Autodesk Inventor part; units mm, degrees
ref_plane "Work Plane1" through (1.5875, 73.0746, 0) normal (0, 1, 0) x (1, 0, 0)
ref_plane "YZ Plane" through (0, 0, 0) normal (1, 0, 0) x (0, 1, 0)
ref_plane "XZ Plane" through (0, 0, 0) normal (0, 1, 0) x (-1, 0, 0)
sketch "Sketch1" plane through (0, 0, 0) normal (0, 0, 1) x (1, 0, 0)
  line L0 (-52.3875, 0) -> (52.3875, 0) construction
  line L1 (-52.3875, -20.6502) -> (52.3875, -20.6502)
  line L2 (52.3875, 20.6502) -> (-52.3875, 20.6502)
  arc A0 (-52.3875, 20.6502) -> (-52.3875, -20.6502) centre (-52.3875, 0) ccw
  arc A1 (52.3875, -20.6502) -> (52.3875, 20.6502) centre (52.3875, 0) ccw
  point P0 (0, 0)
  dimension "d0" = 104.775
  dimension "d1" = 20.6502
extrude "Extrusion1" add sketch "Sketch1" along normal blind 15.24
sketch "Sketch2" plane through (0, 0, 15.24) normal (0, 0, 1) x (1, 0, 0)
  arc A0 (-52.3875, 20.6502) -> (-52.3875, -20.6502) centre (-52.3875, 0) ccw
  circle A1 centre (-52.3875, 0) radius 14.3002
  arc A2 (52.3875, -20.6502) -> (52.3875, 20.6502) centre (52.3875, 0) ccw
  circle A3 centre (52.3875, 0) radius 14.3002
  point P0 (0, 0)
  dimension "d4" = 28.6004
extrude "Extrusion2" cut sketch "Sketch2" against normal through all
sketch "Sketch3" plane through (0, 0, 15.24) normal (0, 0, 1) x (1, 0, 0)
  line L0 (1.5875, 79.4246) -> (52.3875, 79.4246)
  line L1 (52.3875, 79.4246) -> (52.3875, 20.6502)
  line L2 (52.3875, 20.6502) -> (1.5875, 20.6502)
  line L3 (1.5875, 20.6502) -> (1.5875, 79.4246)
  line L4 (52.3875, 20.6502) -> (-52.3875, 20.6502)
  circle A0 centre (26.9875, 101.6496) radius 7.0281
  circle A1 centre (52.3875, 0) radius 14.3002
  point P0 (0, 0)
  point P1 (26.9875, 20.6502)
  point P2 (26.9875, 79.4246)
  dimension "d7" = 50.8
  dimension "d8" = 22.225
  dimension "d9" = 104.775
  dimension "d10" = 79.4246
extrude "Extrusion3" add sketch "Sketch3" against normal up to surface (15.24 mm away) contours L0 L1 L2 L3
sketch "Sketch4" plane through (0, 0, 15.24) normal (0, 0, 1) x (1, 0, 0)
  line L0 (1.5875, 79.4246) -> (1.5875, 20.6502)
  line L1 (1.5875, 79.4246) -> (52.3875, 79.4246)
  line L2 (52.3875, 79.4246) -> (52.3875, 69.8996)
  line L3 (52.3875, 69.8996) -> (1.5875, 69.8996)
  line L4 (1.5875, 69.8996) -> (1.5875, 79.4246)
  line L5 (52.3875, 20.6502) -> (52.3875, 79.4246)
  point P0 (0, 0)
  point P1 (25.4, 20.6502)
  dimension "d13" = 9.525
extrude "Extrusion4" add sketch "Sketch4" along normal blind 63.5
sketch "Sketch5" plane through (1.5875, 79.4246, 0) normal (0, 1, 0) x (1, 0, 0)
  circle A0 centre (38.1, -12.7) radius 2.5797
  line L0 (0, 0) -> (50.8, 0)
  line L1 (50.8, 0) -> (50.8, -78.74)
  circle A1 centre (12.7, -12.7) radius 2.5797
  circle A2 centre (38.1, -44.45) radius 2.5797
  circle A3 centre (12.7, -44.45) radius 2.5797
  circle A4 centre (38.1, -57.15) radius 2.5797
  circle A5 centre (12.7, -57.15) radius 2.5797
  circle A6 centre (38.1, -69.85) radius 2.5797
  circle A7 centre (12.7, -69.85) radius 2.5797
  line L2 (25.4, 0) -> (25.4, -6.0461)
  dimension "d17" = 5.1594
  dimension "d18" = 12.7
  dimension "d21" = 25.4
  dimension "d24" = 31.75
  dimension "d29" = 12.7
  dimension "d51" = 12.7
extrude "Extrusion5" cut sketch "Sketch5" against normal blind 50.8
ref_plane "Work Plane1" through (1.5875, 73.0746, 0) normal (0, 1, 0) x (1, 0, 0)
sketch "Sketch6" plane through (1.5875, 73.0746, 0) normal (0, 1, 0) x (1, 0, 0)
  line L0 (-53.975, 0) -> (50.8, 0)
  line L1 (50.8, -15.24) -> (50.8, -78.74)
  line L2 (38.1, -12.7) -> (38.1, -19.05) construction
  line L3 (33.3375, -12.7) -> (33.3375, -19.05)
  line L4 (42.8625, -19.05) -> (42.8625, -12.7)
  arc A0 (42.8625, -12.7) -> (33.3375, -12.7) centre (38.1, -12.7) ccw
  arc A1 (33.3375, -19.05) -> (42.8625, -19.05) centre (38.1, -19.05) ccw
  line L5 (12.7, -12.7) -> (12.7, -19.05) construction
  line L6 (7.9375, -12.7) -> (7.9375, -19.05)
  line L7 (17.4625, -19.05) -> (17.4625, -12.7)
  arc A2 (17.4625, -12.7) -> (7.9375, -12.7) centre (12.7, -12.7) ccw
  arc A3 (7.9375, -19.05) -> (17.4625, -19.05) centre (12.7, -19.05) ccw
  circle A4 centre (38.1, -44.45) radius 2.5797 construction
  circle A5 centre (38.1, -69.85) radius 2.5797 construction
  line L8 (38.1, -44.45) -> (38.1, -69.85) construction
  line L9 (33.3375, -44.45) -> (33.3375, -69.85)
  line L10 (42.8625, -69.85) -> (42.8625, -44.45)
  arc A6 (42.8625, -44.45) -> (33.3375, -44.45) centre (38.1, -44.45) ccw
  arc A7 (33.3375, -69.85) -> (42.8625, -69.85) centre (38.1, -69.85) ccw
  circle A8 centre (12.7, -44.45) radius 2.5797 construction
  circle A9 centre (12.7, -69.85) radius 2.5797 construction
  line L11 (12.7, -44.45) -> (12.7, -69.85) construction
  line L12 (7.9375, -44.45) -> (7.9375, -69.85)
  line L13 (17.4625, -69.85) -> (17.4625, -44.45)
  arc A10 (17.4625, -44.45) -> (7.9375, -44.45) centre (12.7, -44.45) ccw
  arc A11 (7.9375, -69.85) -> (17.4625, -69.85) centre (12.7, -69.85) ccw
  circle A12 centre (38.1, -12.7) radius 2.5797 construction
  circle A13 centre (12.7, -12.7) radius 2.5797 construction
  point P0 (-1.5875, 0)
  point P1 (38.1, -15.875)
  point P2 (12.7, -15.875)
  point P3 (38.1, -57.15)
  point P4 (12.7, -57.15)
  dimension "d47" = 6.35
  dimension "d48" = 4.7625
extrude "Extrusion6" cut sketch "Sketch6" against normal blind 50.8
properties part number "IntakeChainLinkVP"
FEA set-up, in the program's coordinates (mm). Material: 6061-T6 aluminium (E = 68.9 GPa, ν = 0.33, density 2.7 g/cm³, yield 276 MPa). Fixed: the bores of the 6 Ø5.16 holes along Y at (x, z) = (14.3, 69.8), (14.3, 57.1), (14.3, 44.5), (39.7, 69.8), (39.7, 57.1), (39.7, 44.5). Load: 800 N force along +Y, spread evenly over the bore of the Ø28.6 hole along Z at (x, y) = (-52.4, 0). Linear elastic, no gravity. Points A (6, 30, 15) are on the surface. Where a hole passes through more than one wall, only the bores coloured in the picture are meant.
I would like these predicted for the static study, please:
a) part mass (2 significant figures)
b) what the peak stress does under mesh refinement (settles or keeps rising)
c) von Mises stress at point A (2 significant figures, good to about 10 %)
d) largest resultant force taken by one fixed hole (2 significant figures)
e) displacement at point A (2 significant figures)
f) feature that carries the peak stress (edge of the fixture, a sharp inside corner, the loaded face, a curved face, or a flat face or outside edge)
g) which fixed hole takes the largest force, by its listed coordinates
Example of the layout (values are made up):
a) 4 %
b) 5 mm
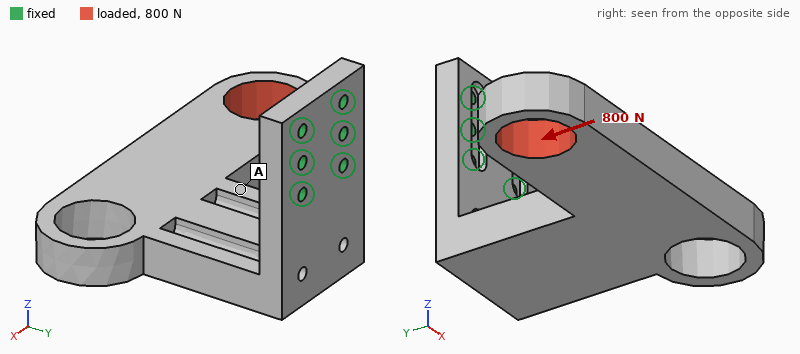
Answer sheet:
a) 360 g
b) keeps rising
c) 16 MPa
d) 3.3 kN
e) 0.30 mm
f) edge of the fixture
g) (14.3, 44.5)
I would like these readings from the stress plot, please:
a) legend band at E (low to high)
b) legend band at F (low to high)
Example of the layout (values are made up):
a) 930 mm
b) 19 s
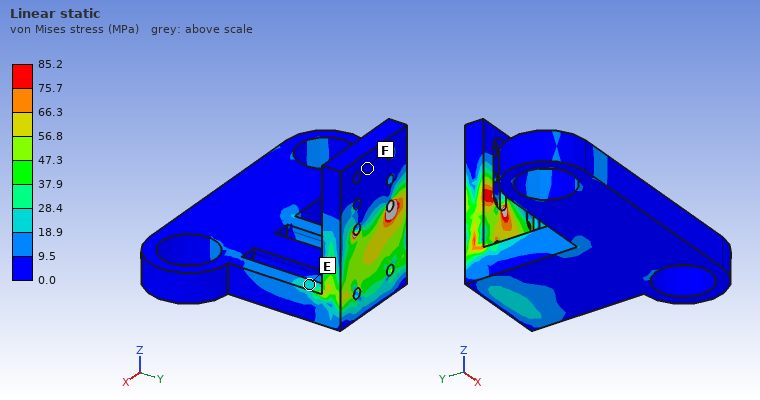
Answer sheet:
a) 18.9 to 28.4 MPa
b) 0.0 to 9.5 MPa
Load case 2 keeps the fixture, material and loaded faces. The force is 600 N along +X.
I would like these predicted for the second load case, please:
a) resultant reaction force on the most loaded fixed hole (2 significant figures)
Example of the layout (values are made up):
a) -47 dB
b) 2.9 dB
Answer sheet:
a) 1.9 kN
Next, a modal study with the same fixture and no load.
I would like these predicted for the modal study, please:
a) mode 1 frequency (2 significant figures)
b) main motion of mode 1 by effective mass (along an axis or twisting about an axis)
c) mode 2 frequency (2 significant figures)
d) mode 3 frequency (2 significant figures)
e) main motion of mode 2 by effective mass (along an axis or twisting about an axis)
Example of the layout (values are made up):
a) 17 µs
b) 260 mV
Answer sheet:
a) 320 Hz
b) along Z
c) 480 Hz
d) 1000 Hz
e) along X
